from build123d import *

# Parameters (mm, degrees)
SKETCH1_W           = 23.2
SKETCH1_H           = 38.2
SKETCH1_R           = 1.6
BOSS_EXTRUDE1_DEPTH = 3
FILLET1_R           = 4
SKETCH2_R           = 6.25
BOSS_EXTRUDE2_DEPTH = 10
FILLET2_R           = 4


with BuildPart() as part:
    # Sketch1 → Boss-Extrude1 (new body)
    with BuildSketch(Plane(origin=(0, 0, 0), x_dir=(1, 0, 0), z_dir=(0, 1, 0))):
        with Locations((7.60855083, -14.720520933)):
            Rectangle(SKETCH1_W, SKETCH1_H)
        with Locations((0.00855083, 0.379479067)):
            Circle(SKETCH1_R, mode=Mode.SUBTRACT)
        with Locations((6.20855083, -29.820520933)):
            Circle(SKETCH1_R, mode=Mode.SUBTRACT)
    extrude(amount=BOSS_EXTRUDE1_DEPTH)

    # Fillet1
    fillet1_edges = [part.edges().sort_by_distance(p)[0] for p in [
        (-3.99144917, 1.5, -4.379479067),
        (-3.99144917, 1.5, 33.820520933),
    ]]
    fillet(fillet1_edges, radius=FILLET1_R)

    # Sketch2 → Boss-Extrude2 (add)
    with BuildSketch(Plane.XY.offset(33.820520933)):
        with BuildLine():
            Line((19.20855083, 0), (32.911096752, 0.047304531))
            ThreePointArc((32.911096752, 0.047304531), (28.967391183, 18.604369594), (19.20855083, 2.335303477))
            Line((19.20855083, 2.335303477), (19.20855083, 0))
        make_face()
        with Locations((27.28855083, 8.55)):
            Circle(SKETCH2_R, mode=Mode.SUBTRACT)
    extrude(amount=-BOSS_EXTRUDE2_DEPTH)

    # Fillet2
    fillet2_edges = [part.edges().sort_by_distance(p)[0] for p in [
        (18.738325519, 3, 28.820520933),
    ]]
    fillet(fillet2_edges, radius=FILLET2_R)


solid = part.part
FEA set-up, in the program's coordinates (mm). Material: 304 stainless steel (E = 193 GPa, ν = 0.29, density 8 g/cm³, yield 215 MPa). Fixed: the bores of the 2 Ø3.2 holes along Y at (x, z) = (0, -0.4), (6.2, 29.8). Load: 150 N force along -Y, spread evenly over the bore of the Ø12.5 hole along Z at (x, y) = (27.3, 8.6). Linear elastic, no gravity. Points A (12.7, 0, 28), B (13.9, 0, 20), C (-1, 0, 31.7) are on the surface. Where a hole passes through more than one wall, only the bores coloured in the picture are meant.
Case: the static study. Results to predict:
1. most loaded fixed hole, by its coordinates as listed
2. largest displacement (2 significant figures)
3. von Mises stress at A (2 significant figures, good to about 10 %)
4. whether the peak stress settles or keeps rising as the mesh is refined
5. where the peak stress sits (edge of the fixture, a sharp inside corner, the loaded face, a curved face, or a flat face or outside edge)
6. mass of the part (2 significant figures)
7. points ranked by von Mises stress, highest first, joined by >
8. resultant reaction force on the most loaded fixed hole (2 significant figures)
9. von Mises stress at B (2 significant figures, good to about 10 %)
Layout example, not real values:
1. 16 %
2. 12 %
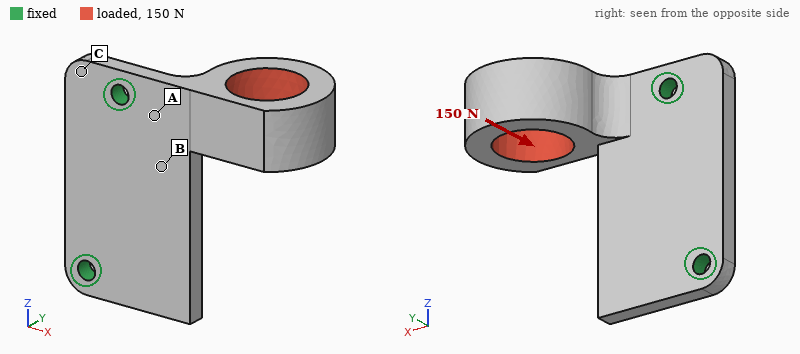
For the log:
1. (6.2, 29.8)
2. 96 µm
3. 81 MPa
4. keeps rising
5. edge of the fixture
6. 37 g
7. A > B > C
8. 160 N
9. 54 MPa
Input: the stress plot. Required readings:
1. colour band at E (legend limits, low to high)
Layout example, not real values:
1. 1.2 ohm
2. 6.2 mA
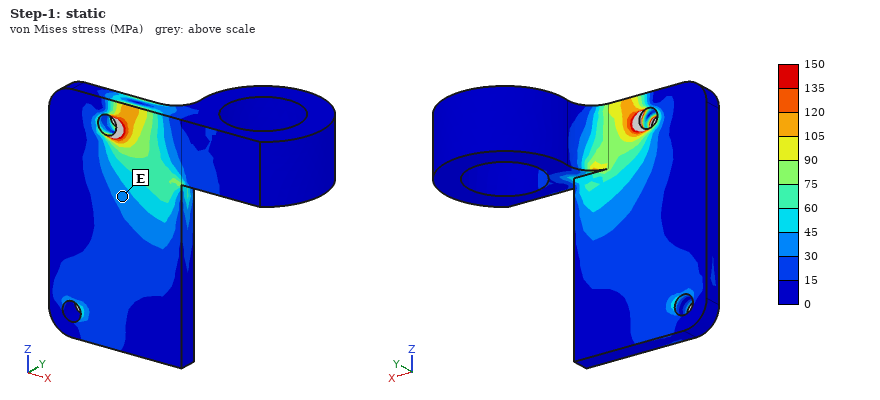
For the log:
1. 30 to 45 MPa
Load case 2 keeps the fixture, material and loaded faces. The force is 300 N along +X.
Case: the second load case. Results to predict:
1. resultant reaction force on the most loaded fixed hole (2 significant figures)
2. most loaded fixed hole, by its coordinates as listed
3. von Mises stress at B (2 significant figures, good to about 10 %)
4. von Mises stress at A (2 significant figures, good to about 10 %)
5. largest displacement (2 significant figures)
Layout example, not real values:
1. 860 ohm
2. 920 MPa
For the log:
1. 290 N
2. (6.2, 29.8)
3. 49 MPa
4. 71 MPa
5. 86 µm
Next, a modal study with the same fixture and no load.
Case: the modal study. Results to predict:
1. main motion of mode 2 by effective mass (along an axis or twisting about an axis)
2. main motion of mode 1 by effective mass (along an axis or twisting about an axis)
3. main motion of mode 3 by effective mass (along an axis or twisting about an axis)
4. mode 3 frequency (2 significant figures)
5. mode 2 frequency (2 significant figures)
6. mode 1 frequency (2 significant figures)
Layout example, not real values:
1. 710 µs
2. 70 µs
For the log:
1. along Z
2. along Y
3. along Y
4. 7900 Hz
5. 4000 Hz
6. 1700 Hz
